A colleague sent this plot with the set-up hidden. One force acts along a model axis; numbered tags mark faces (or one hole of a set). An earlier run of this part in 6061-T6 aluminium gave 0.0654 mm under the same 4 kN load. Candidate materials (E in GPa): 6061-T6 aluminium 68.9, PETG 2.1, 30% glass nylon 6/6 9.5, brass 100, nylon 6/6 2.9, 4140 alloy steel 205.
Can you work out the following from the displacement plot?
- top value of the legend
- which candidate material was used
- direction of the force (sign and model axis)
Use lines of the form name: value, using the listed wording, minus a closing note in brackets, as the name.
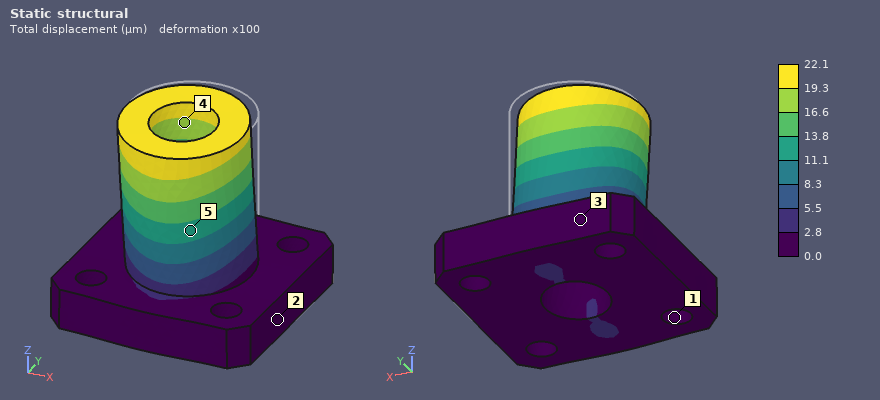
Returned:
top value of the legend: 22.1 µm
which candidate material was used: 4140 alloy steel
direction of the force: -Y
